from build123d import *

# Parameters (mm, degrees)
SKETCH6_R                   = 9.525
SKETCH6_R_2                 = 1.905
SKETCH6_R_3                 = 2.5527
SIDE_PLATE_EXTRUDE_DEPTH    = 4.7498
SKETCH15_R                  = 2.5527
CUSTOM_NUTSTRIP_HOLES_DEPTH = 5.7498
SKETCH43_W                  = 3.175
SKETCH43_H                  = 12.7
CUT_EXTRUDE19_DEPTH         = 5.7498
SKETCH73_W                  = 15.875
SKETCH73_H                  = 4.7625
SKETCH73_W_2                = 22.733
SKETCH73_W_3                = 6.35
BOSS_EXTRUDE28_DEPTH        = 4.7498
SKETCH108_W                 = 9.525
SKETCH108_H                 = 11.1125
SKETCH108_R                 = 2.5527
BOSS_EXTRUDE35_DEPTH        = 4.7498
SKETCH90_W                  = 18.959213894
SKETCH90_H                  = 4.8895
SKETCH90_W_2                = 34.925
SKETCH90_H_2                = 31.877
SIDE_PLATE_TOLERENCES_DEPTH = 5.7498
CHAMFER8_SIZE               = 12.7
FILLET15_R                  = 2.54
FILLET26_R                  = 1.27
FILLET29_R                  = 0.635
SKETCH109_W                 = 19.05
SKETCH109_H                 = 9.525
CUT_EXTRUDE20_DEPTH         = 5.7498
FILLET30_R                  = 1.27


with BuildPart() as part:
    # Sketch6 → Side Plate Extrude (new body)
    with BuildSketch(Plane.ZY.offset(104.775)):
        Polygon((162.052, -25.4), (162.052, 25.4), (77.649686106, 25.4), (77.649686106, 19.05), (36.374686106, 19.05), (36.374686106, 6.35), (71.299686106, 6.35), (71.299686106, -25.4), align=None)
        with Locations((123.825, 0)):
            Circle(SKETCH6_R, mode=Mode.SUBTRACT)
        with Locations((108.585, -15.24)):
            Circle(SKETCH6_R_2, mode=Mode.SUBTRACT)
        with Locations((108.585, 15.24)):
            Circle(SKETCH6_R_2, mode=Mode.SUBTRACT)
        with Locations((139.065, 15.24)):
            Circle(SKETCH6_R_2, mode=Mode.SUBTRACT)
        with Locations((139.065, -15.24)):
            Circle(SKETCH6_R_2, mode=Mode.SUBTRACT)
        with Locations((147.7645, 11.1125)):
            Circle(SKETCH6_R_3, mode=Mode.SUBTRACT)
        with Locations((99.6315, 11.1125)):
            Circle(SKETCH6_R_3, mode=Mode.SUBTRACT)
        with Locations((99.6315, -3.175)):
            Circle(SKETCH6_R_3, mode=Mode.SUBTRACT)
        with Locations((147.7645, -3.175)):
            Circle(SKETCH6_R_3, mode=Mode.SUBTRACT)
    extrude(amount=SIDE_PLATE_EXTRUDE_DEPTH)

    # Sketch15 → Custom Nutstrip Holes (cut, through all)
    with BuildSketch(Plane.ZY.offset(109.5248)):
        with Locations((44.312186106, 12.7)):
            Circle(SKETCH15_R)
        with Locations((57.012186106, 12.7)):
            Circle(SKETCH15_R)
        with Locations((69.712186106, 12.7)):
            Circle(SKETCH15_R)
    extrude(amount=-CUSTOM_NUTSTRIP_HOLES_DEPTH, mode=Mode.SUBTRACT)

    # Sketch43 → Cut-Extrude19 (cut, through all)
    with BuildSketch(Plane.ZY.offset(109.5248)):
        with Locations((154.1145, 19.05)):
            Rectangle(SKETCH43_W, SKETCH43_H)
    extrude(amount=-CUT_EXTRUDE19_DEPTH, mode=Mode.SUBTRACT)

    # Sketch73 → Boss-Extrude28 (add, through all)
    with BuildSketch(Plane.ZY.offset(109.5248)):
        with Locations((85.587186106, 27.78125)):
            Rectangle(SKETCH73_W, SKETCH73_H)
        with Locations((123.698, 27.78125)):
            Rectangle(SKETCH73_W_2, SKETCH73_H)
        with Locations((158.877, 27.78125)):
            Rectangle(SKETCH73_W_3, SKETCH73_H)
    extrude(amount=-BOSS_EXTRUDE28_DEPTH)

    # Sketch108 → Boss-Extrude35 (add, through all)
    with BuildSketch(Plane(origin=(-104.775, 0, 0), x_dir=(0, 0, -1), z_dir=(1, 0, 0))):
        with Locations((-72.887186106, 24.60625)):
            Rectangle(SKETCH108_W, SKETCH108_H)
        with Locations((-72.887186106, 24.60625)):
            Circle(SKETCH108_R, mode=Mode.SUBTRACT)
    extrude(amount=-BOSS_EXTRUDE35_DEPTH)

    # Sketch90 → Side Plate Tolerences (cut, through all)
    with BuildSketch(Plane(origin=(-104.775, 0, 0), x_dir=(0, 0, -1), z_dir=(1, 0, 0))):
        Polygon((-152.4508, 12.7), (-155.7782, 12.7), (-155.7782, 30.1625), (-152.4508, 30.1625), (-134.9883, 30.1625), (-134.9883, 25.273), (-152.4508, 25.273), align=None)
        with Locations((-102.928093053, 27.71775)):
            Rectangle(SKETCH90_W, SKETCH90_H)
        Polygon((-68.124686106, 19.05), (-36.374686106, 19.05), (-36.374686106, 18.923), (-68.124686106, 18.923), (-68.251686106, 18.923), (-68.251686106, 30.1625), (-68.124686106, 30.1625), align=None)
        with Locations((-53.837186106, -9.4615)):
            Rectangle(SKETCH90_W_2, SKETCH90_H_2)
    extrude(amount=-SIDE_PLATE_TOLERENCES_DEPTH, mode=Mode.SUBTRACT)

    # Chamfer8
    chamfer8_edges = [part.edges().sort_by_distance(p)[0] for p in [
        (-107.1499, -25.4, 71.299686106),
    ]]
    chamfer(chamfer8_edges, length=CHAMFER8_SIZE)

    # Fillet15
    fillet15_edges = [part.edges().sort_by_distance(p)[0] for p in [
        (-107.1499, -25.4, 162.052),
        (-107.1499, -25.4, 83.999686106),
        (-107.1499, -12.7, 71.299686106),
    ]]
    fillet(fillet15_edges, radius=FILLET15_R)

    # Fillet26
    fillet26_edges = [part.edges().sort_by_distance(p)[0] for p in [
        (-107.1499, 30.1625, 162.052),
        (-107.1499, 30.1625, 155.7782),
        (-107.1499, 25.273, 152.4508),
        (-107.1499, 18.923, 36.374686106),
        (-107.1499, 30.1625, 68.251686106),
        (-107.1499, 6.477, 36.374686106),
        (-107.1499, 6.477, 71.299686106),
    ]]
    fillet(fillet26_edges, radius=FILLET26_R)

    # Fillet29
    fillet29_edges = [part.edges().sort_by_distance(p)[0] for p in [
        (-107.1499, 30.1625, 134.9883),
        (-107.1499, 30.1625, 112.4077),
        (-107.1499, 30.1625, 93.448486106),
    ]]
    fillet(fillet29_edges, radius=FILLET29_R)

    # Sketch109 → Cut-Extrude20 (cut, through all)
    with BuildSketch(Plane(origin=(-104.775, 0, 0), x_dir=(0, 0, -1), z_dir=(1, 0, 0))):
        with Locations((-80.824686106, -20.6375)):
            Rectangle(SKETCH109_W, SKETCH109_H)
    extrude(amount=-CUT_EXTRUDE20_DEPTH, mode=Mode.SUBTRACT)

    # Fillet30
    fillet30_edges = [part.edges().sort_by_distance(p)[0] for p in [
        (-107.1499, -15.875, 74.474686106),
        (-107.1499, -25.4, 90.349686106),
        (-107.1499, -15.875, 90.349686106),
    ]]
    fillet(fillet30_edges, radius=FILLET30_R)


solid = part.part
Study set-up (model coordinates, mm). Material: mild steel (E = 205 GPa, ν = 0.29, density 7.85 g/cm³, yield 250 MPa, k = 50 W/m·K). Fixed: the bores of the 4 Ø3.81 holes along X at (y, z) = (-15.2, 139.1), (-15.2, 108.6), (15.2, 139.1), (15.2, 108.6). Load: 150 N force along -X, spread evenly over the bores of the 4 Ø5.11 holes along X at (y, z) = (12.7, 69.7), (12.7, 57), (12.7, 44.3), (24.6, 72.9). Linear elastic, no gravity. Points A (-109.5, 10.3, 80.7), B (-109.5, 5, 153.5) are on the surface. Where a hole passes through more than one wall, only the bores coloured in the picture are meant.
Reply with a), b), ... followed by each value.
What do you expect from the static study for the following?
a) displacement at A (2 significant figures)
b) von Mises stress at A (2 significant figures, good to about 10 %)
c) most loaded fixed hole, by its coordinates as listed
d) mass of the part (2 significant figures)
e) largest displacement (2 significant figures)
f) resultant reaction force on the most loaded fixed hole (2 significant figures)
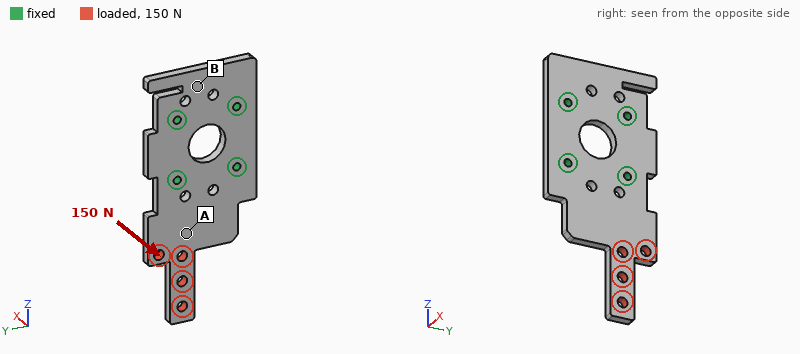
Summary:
a) 0.035 mm
b) 26 MPa
c) (15.2, 108.6)
d) 170 g
e) 0.18 mm
f) 180 N
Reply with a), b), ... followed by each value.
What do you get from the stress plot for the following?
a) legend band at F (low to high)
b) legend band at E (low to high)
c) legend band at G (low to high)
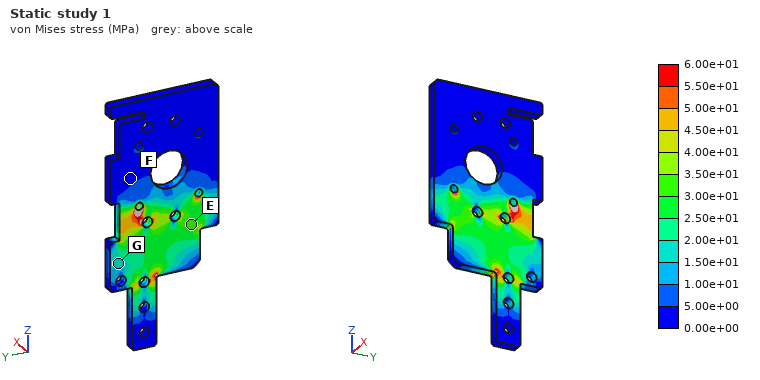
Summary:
a) 0.00e+00 to 5.00e+00 MPa
b) 3.00e+01 to 3.50e+01 MPa
c) 1.50e+01 to 2.00e+01 MPa
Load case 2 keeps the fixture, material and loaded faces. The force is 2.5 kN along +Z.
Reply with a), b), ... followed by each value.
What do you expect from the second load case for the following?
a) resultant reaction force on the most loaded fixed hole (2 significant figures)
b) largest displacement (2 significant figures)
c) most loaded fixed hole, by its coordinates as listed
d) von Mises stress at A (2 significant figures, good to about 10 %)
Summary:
a) 2.0 kN
b) 12 µm
c) (15.2, 108.6)
d) 21 MPa
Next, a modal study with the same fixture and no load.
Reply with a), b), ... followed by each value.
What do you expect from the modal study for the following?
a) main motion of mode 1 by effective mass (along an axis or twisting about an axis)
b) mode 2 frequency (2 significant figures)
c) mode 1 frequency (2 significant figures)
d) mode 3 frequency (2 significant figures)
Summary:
a) along X
b) 3900 Hz
c) 1200 Hz
d) 5100 Hz
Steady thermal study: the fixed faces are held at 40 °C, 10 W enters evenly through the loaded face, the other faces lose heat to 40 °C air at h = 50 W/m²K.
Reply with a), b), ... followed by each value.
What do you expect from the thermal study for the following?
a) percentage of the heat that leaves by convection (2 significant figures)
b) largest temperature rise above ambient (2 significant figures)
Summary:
a) 52 %
b) 55 K
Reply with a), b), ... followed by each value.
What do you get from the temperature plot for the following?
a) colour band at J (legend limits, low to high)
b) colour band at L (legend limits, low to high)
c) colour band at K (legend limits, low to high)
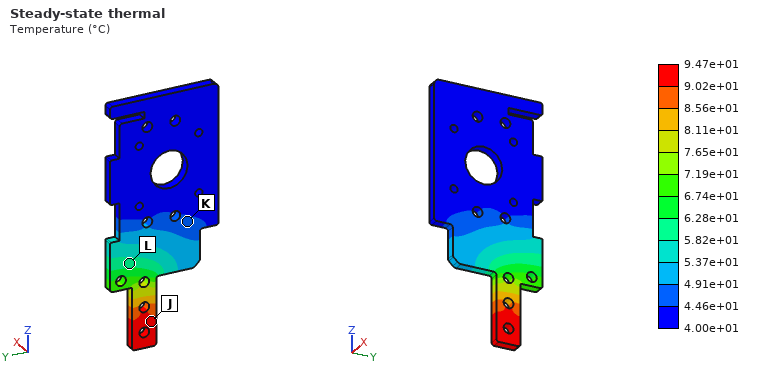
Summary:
a) 9.02e+01 to 9.47e+01 °C
b) 5.82e+01 to 6.28e+01 °C
c) 4.46e+01 to 4.91e+01 °C
